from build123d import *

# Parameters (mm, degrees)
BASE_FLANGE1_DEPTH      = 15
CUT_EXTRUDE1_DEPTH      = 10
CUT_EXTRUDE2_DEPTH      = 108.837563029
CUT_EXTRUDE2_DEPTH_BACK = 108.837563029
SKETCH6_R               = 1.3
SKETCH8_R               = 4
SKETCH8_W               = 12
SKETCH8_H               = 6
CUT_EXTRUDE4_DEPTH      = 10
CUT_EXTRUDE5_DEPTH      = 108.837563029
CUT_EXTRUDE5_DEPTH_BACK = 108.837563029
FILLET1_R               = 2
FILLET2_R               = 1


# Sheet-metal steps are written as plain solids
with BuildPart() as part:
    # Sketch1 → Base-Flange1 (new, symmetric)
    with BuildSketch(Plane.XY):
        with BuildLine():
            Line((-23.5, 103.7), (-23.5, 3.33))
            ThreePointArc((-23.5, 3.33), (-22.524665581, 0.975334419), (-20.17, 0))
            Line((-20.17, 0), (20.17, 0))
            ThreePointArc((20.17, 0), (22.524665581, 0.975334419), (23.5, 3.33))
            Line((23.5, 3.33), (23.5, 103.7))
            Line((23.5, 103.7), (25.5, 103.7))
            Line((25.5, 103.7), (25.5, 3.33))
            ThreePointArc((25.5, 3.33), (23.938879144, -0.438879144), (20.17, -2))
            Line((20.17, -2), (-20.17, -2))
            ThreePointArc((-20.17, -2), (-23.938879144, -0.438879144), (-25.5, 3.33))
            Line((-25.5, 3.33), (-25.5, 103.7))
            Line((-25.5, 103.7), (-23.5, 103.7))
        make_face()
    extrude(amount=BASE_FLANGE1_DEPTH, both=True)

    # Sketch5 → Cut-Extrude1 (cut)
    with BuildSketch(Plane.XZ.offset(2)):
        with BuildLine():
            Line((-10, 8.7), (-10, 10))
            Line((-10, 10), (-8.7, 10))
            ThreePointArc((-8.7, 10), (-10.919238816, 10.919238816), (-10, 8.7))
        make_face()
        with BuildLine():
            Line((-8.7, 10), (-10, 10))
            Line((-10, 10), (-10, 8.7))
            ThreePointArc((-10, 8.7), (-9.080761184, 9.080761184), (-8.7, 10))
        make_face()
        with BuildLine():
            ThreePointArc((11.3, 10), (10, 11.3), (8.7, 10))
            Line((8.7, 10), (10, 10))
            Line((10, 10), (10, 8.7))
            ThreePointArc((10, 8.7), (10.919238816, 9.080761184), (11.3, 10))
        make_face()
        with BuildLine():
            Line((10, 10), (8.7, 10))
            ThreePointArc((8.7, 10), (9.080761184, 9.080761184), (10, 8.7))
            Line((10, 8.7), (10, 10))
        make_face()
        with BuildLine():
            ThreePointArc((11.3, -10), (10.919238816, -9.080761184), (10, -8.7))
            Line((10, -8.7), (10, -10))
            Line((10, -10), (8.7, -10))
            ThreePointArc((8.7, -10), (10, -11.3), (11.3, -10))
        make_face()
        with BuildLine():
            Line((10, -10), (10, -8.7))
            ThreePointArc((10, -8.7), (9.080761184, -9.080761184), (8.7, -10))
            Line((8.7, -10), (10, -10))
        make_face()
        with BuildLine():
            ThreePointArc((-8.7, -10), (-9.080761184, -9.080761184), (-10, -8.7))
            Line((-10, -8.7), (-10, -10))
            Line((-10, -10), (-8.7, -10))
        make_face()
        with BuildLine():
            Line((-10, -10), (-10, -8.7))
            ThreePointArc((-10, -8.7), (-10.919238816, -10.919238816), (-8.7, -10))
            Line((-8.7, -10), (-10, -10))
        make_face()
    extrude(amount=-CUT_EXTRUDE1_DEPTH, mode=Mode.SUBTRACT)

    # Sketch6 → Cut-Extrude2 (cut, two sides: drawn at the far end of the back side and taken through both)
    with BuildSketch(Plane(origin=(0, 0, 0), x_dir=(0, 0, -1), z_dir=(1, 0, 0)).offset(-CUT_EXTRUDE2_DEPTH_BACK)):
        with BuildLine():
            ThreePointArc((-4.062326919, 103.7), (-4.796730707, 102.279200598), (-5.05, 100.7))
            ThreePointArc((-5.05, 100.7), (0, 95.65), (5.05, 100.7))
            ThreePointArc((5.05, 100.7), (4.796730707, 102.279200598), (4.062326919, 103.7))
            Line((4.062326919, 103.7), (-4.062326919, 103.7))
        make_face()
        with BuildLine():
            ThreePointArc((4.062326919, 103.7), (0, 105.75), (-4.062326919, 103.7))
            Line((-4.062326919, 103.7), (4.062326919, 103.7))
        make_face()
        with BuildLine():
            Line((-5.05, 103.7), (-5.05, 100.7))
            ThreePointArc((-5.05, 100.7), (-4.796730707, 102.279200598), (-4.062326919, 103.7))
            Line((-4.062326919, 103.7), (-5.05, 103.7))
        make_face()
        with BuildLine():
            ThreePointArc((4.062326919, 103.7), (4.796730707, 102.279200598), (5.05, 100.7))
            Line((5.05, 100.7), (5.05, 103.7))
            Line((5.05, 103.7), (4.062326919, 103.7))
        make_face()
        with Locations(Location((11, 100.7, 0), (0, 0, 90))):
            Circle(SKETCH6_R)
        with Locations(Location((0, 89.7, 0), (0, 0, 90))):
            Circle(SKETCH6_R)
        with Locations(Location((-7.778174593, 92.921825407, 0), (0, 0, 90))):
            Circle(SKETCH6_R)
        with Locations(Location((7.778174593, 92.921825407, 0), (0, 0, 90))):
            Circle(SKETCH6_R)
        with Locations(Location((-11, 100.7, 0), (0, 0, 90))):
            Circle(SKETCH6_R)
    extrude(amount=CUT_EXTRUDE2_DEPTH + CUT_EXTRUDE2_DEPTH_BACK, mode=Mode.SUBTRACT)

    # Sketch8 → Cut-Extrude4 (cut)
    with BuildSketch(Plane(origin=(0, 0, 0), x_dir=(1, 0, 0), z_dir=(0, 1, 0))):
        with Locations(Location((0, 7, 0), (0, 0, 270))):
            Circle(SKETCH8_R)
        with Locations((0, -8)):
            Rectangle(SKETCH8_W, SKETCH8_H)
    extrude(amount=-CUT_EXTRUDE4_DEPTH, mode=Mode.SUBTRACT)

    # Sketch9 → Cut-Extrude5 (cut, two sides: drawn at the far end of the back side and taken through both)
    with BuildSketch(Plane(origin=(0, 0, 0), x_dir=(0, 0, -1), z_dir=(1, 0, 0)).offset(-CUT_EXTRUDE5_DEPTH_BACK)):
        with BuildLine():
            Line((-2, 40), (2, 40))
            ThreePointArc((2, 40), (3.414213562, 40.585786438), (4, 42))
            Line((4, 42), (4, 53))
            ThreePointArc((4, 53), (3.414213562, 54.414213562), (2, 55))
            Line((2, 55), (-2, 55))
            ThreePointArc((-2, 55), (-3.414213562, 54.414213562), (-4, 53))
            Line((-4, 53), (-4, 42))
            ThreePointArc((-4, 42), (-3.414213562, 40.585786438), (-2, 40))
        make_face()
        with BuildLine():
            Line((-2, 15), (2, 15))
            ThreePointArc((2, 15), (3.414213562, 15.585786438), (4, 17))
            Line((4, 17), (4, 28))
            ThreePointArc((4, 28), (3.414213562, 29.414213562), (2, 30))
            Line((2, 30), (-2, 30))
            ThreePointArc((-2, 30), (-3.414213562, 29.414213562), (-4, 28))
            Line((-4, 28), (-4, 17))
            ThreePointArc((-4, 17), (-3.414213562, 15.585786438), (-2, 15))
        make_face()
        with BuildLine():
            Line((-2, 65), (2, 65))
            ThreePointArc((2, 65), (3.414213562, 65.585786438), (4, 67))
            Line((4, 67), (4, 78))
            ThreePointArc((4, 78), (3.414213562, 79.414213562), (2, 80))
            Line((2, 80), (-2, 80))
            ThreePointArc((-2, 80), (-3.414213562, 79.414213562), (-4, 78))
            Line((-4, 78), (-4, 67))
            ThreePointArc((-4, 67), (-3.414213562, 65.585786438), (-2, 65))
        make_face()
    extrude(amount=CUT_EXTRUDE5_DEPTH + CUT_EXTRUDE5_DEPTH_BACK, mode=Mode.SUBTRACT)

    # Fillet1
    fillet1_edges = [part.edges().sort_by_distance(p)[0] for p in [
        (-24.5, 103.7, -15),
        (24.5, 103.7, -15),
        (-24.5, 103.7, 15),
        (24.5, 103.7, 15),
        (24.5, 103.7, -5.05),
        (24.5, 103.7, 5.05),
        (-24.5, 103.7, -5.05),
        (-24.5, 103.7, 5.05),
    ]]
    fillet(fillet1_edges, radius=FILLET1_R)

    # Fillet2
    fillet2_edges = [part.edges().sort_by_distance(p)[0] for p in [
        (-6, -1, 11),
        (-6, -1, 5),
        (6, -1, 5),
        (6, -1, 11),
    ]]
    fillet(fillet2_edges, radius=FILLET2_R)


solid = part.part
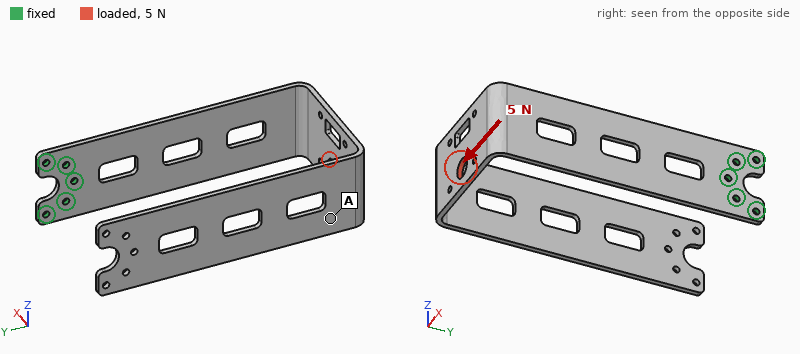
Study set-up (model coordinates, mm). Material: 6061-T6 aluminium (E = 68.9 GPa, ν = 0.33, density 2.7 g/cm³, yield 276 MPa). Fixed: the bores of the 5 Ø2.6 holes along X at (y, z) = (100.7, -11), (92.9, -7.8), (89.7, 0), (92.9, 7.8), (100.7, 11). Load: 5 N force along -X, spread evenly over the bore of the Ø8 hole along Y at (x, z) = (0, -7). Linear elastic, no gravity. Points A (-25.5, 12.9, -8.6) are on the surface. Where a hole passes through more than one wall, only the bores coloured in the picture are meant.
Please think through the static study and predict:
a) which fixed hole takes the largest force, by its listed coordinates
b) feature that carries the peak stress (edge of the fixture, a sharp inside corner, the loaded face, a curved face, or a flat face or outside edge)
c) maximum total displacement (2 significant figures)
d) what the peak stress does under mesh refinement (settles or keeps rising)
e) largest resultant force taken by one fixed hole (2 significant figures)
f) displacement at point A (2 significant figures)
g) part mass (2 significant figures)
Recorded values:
(89.7, 0)
edge of the fixture
1.4 mm
keeps rising
30 N
1.3 mm
36 g
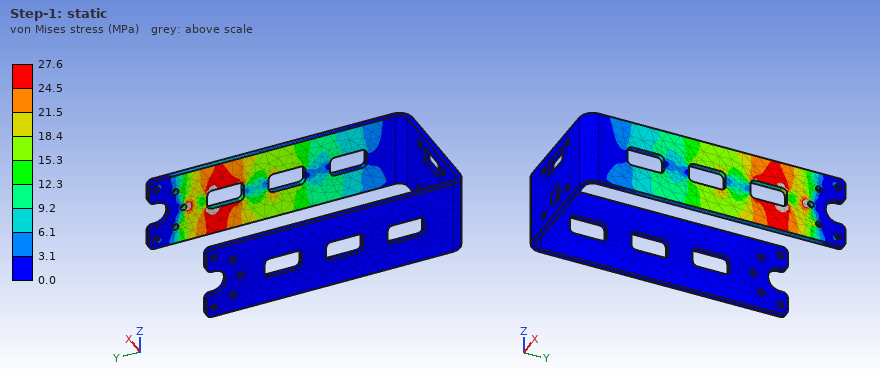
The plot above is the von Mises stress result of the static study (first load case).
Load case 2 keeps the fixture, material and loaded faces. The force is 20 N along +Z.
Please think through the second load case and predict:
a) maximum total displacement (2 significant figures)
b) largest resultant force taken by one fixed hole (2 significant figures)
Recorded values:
1.4 mm
67 N
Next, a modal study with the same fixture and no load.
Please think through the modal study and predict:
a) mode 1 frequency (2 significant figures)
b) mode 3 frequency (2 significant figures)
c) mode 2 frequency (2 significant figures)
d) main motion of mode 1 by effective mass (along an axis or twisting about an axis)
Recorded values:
60 Hz
88 Hz
87 Hz
along Y
